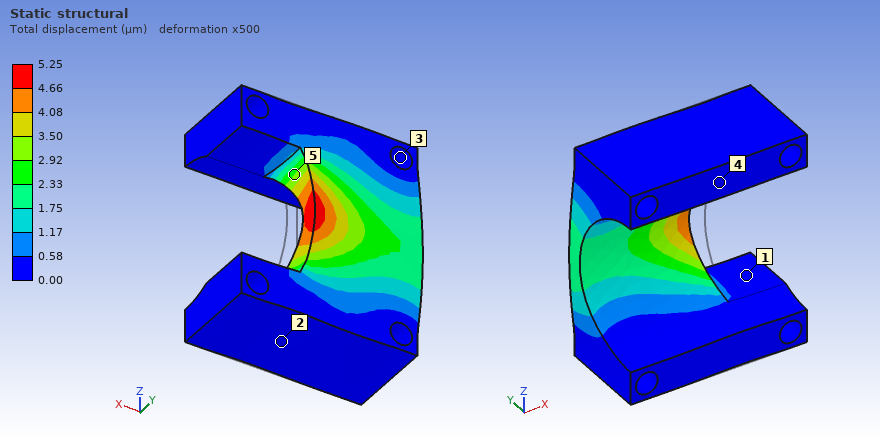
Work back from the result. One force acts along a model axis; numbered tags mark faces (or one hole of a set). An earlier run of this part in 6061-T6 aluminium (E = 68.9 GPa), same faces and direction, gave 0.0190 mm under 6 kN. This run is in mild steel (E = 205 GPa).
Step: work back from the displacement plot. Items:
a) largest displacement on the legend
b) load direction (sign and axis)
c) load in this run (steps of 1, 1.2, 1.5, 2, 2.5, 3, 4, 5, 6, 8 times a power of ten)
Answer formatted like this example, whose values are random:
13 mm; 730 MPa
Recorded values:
5.25 µm; -X; 5 kN
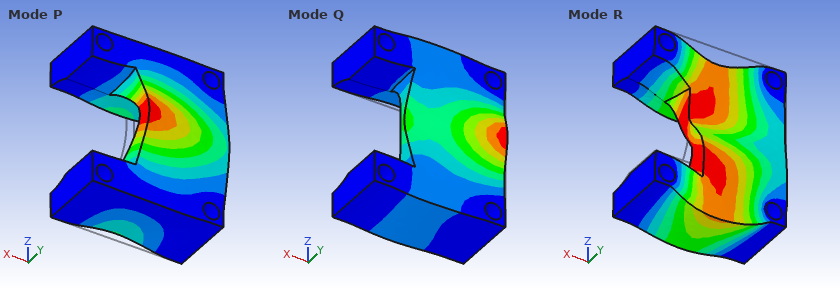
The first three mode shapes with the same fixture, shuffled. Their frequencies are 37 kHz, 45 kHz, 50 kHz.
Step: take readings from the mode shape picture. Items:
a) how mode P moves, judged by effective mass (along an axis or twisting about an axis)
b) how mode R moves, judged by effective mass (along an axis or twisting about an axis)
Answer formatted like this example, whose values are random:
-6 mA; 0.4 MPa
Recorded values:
along Y; along Z
